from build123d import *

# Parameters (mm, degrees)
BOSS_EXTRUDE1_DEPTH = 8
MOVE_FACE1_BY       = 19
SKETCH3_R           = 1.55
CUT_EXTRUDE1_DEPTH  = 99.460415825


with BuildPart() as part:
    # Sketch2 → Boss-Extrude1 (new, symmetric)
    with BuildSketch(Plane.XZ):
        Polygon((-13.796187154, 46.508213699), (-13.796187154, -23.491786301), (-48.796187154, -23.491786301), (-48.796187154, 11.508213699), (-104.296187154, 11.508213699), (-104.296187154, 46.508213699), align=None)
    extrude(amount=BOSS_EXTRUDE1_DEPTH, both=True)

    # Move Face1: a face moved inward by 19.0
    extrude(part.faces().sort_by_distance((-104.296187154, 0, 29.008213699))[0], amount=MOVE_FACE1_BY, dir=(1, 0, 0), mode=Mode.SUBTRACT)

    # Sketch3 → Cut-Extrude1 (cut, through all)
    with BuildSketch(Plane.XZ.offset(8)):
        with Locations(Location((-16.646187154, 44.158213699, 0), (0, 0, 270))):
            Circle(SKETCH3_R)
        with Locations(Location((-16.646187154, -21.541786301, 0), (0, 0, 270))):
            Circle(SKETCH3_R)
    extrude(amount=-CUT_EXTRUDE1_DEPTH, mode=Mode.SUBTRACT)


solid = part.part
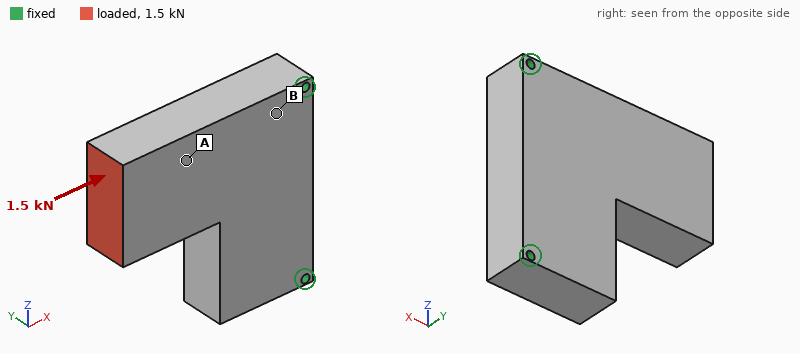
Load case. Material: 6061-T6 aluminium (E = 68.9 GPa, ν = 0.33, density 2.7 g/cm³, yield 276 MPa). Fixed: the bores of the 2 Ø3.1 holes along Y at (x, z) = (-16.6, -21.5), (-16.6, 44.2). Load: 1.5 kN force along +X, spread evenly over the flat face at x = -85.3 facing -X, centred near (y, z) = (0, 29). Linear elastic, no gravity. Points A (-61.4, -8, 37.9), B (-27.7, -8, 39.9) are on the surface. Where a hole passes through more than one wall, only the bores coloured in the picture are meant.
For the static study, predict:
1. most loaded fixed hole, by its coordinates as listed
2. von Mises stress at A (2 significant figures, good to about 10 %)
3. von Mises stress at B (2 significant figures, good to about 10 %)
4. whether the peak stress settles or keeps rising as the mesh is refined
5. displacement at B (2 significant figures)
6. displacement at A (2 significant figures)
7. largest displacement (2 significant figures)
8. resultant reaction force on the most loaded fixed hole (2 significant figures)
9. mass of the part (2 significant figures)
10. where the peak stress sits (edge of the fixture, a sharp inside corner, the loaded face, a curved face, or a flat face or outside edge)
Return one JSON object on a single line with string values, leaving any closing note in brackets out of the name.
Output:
{"most loaded fixed hole, by its coordinates as listed": "(-16.6, 44.2)", "von Mises stress at A": "2.7 MPa", "von Mises stress at B": "5.2 MPa", "whether the peak stress settles or keeps rising as the mesh is refined": "keeps rising", "displacement at B": "1.4 µm", "displacement at A": "3.0 µm", "largest displacement": "4.0 µm", "resultant reaction force on the most loaded fixed hole": "1.2 kN", "mass of the part": "160 g", "where the peak stress sits": "edge of the fixture"}
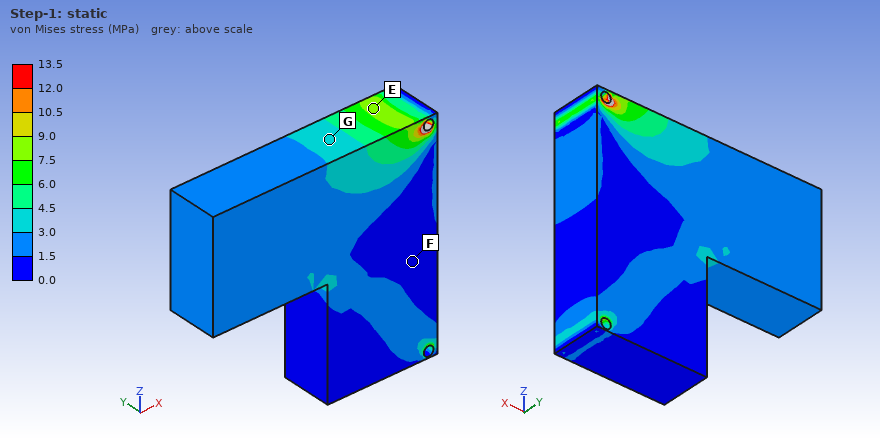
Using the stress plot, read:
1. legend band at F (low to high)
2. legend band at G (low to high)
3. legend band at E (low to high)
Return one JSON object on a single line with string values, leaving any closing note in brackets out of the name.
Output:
{"legend band at F": "0.0 to 1.5 MPa", "legend band at G": "3.0 to 4.5 MPa", "legend band at E": "7.5 to 9.0 MPa"}
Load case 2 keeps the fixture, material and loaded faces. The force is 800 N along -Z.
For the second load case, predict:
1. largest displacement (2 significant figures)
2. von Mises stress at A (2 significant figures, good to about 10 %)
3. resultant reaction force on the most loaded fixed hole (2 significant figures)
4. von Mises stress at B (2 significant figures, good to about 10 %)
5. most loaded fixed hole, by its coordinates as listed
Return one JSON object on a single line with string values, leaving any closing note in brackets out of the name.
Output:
{"largest displacement": "17 µm", "von Mises stress at A": "3.9 MPa", "resultant reaction force on the most loaded fixed hole": "1.1 kN", "von Mises stress at B": "4.1 MPa", "most loaded fixed hole, by its coordinates as listed": "(-16.6, -21.5)"}
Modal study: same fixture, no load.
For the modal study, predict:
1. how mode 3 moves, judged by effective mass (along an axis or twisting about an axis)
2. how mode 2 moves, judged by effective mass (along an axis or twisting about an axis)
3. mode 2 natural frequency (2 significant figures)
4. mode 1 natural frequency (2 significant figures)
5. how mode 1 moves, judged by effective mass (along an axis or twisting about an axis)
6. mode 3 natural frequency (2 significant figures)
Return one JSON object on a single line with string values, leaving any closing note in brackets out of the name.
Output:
{"how mode 3 moves, judged by effective mass": "along Y", "how mode 2 moves, judged by effective mass": "along Z", "mode 2 natural frequency": "7000 Hz", "mode 1 natural frequency": "2100 Hz", "how mode 1 moves, judged by effective mass": "along Y", "mode 3 natural frequency": "7800 Hz"}
